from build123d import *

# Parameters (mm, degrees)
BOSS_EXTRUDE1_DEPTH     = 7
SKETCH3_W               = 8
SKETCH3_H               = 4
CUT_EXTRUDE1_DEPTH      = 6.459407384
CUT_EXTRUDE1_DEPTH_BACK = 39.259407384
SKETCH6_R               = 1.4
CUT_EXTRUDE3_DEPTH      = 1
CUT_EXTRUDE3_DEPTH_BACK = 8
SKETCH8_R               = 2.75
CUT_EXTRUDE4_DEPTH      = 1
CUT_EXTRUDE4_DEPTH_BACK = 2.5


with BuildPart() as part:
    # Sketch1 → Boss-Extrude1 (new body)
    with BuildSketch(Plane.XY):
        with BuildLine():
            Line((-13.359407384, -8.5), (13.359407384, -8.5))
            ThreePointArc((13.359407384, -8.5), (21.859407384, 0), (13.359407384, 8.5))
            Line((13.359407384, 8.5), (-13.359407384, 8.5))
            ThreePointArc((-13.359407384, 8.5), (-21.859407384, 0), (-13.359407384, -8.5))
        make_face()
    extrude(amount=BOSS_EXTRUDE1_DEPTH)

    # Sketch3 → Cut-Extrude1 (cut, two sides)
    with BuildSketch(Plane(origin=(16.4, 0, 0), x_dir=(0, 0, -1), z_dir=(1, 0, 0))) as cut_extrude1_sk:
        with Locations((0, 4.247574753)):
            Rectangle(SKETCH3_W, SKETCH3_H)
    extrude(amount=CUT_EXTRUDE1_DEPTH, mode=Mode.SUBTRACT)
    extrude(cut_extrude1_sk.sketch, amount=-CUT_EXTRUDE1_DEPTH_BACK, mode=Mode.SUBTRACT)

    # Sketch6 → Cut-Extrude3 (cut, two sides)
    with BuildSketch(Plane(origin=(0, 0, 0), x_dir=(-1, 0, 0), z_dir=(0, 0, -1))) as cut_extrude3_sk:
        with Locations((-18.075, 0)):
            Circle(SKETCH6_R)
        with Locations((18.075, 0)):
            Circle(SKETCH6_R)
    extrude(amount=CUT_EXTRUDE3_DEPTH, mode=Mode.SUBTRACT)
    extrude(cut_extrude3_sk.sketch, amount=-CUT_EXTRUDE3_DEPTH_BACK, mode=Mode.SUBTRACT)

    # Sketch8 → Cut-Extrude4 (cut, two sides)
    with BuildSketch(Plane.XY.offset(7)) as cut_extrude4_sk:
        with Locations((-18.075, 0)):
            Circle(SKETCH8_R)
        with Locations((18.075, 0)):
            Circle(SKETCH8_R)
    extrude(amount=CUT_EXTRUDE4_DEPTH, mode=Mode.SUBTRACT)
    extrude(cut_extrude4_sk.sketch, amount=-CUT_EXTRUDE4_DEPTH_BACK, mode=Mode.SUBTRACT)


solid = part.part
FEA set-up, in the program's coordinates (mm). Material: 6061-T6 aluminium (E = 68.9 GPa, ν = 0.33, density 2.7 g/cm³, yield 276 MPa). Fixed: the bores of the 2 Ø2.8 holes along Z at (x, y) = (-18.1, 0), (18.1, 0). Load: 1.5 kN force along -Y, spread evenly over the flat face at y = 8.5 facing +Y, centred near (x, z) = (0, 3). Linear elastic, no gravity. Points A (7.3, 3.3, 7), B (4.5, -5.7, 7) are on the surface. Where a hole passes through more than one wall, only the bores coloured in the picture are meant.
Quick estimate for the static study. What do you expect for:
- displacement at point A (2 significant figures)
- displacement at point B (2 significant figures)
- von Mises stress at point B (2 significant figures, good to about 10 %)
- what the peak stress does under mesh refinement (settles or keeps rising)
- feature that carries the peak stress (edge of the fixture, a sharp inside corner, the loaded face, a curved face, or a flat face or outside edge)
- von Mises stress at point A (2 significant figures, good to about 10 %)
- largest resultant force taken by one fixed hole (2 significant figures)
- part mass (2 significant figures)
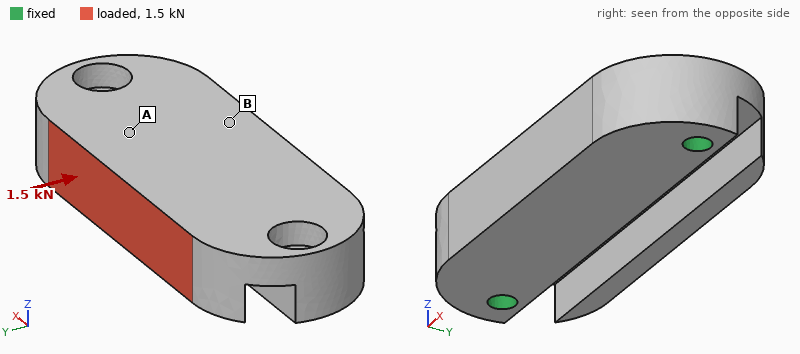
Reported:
8.7 µm
11 µm
17 MPa
keeps rising
edge of the fixture
38 MPa
760 N
11 g
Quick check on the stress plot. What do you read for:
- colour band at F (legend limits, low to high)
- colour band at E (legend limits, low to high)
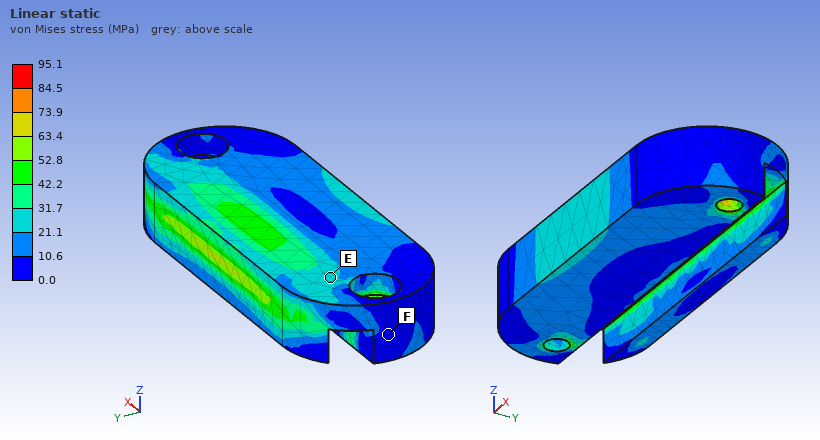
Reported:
0.0 to 10.6 MPa
21.1 to 31.7 MPa
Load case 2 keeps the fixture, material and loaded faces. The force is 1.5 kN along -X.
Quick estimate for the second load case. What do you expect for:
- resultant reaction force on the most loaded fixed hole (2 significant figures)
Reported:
830 N
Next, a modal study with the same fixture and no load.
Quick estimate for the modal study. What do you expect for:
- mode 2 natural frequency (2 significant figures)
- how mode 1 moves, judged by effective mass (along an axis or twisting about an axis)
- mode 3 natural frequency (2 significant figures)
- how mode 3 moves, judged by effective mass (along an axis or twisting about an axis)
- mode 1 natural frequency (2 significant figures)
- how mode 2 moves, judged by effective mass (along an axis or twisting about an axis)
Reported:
16 kHz
along Z
22 kHz
along Y
14 kHz
along Z
